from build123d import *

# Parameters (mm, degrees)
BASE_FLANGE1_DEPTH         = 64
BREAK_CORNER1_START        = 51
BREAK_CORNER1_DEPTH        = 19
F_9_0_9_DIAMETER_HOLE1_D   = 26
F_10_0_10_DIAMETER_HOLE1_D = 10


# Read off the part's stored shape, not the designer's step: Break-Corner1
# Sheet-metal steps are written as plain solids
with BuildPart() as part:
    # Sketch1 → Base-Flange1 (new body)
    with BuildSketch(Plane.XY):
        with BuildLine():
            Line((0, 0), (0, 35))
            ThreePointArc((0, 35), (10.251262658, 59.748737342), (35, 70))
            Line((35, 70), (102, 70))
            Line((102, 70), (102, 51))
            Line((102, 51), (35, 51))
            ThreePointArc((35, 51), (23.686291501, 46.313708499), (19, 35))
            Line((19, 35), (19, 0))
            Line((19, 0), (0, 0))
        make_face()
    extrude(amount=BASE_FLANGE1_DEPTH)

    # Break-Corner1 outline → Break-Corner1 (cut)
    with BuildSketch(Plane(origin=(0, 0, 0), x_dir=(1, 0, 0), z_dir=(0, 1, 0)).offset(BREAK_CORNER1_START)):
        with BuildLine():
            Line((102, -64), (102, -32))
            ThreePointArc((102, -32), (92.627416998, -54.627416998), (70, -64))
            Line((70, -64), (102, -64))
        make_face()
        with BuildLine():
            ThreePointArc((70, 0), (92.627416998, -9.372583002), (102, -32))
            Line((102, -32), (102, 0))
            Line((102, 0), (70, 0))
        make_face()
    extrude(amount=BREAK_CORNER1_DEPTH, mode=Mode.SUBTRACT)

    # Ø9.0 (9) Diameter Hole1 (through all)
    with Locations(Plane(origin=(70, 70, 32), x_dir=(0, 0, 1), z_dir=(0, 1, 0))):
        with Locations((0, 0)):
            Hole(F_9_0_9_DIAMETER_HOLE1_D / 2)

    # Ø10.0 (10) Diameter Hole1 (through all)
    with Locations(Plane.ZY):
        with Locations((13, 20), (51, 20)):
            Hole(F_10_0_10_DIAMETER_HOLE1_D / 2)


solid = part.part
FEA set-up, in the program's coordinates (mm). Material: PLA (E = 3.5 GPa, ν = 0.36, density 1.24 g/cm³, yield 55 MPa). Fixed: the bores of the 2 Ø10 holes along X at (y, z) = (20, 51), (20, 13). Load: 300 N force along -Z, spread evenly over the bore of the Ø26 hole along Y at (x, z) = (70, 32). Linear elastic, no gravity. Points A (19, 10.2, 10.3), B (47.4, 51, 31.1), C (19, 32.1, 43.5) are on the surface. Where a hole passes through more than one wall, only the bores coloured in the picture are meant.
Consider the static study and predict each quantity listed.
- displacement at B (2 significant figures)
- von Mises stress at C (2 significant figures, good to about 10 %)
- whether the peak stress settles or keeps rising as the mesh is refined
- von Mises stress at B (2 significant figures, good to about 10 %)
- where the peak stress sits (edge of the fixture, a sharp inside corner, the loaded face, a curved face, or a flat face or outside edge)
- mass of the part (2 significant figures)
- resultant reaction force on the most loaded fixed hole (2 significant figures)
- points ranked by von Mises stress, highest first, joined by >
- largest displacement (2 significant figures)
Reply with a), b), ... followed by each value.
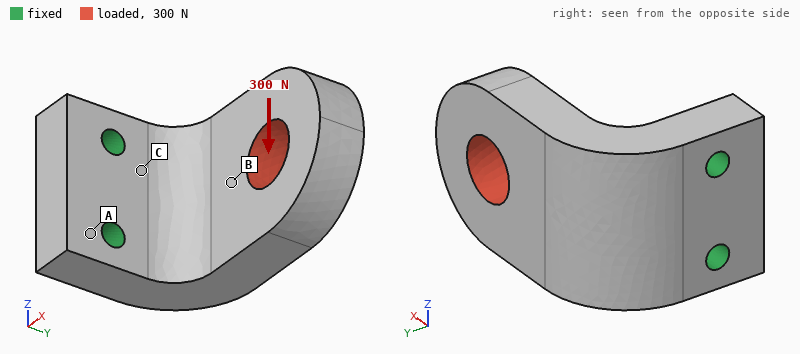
a) 0.096 mm
b) 2.7 MPa
c) keeps rising
d) 1.5 MPa
e) edge of the fixture
f) 190 g
g) 480 N
h) C > B > A
i) 0.24 mm
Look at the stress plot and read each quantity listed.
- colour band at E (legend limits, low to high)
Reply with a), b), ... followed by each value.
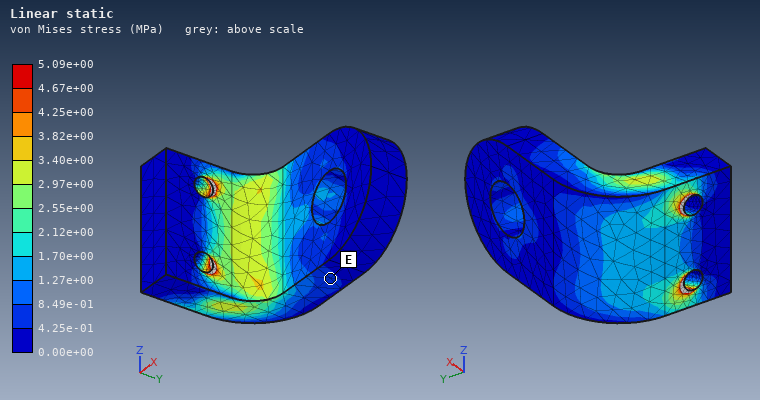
a) 4.25e-01 to 8.49e-01 MPa
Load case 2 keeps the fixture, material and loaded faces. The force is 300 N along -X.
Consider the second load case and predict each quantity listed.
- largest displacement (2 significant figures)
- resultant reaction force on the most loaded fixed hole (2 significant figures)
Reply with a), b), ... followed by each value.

a) 0.20 mm
b) 150 N
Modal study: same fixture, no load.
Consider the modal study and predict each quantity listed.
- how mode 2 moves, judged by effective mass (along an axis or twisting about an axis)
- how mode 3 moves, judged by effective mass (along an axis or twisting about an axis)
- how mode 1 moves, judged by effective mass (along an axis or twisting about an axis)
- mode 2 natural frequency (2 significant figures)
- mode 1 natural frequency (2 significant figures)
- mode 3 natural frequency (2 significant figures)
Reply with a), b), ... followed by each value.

a) along Z
b) along X
c) along Y
d) 760 Hz
e) 460 Hz
f) 1600 Hz
